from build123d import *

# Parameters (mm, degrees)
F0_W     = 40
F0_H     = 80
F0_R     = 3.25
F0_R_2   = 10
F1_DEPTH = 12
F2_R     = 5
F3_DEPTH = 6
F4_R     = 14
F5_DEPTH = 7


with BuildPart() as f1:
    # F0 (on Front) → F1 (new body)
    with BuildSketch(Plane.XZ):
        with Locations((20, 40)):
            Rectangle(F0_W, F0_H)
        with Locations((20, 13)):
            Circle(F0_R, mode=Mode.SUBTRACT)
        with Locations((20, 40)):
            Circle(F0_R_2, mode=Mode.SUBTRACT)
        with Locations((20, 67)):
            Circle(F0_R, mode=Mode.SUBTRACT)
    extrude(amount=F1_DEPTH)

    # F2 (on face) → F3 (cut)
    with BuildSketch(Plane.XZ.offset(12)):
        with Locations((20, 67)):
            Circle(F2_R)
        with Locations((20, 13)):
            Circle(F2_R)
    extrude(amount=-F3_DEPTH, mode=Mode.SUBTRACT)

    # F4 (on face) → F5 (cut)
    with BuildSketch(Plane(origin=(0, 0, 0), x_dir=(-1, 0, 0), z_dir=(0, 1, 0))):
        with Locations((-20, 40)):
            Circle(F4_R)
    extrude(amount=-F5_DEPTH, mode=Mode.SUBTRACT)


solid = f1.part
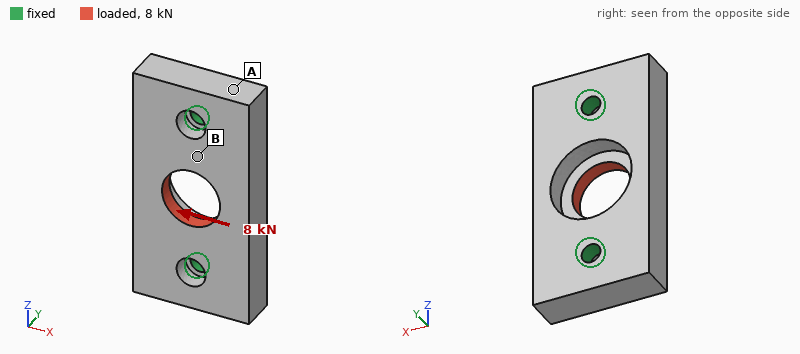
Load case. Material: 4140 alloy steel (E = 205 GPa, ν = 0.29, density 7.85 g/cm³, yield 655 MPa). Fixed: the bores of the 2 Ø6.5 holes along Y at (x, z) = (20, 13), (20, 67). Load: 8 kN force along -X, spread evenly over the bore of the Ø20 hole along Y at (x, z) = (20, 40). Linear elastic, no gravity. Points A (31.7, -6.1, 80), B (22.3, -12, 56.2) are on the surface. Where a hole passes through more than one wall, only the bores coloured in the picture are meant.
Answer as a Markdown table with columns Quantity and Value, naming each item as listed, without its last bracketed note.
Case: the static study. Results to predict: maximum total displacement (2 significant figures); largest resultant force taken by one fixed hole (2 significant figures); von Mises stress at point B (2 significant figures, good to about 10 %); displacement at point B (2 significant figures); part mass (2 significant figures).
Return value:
| Quantity | Value |
|---|---|
| maximum total displacement | 19 µm |
| largest resultant force taken by one fixed hole | 4.0 kN |
| von Mises stress at point B | 40 MPa |
| displacement at point B | 8.6 µm |
| part mass | 240 g |
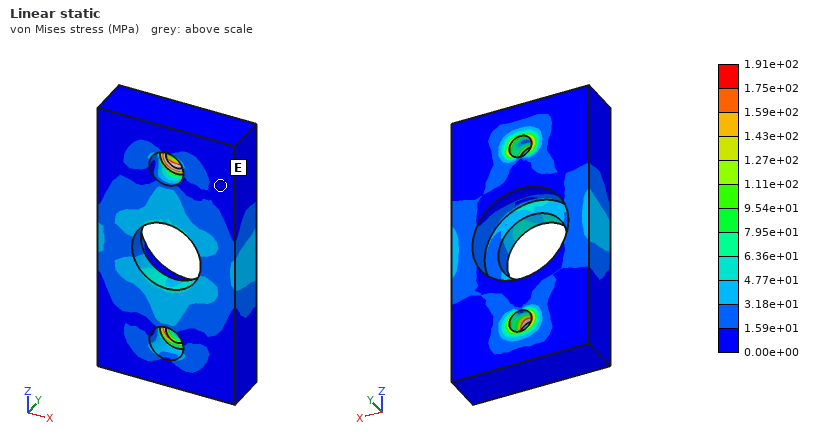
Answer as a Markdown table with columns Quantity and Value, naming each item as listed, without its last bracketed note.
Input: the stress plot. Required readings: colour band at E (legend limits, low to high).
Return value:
| Quantity | Value |
|---|---|
| colour band at E | 0.00e+00 to 1.59e+01 MPa |
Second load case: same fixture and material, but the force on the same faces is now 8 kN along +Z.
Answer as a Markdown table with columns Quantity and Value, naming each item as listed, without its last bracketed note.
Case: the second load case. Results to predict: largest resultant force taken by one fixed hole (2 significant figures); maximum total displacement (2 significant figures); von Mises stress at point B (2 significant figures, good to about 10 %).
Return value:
| Quantity | Value |
|---|---|
| largest resultant force taken by one fixed hole | 4.1 kN |
| maximum total displacement | 4.5 µm |
| von Mises stress at point B | 28 MPa |
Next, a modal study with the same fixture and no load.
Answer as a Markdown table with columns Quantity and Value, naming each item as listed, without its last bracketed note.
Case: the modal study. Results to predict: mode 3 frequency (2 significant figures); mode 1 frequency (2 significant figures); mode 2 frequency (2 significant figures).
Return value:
| Quantity | Value |
|---|---|
| mode 3 frequency | 11 kHz |
| mode 1 frequency | 7200 Hz |
| mode 2 frequency | 11 kHz |
